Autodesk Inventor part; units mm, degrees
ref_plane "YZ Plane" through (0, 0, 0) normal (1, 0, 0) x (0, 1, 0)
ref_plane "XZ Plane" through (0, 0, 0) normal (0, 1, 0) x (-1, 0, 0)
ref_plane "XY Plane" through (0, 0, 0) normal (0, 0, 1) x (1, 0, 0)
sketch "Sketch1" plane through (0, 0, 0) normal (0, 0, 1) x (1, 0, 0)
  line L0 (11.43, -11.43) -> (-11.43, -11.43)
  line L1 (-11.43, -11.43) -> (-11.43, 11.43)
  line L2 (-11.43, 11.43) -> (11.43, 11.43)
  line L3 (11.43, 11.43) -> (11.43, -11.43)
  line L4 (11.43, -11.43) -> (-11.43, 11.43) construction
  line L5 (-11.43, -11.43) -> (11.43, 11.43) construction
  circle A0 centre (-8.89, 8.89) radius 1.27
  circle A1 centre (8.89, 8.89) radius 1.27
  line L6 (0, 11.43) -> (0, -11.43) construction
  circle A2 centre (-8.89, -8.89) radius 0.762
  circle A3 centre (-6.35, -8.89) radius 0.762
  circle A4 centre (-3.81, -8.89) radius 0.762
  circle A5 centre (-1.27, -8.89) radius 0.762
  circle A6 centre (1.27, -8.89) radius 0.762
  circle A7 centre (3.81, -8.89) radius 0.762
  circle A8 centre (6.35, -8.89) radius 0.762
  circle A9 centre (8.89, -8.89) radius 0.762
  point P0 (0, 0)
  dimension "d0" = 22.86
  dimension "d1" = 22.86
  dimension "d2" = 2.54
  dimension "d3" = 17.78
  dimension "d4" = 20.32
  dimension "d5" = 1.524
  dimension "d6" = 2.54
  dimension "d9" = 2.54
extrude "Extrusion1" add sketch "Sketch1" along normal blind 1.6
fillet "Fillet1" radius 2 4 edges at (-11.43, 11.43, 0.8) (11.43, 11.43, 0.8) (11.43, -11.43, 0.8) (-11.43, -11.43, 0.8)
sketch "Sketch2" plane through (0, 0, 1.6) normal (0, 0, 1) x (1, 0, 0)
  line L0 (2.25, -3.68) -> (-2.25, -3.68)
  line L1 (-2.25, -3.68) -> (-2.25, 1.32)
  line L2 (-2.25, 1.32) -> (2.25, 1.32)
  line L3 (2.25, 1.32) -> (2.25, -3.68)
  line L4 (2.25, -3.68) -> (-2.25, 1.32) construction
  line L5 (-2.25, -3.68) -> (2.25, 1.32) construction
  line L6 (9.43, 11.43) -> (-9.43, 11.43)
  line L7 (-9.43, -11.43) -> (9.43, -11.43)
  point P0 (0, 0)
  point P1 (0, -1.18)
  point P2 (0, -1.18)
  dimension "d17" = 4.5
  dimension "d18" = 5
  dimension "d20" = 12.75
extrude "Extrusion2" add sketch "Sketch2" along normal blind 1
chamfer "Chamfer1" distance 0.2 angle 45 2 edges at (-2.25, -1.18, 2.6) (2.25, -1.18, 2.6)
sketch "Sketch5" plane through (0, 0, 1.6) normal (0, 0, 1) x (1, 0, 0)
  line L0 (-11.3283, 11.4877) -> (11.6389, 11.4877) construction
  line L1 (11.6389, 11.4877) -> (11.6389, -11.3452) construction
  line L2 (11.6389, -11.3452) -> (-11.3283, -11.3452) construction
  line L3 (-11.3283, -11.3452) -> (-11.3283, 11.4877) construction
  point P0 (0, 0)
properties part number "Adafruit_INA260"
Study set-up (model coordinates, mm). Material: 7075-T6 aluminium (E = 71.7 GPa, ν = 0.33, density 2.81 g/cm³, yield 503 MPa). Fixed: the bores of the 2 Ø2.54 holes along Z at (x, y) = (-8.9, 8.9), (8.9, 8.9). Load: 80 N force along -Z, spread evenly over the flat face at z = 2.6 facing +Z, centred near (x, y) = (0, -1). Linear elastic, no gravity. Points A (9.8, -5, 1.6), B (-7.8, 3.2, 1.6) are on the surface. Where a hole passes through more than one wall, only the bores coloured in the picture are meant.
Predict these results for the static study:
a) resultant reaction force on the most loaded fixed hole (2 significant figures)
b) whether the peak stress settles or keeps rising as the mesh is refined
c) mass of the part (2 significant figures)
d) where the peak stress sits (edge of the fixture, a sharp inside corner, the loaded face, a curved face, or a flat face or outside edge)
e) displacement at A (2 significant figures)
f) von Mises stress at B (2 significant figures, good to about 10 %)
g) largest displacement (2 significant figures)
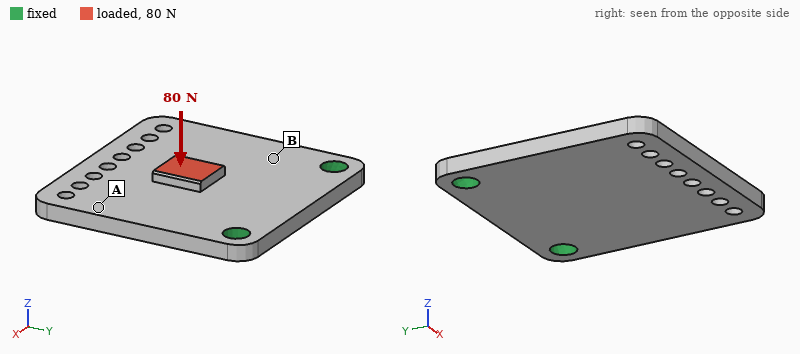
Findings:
40 N
keeps rising
2.3 g
edge of the fixture
0.081 mm
38 MPa
0.15 mm
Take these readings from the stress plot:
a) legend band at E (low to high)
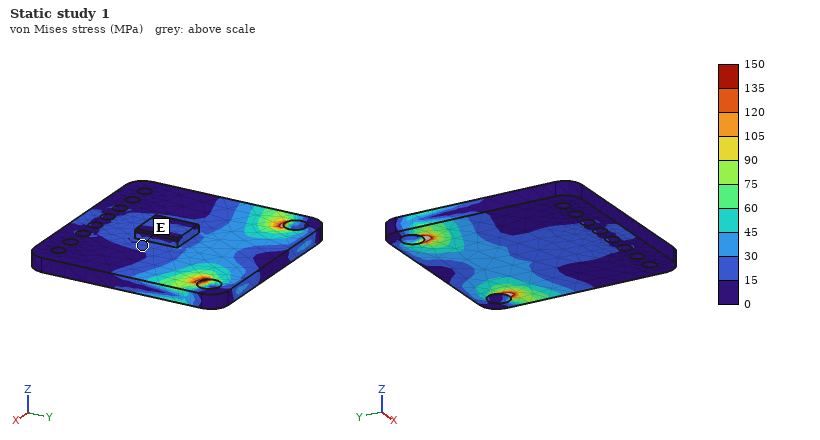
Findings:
15 to 30 MPa
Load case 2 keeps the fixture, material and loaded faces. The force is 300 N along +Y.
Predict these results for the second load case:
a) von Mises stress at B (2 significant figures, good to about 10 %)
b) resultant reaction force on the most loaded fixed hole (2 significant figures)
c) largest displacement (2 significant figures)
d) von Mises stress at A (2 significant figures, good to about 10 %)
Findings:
57 MPa
160 N
0.15 mm
11 MPa
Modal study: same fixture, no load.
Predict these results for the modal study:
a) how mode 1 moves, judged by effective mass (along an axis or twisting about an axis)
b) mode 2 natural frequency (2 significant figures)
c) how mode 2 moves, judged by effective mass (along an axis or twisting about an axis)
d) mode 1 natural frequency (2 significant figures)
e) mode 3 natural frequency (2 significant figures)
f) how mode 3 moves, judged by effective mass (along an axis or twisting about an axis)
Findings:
along Z
7900 Hz
twisting about Y
3200 Hz
19 kHz
along Z
